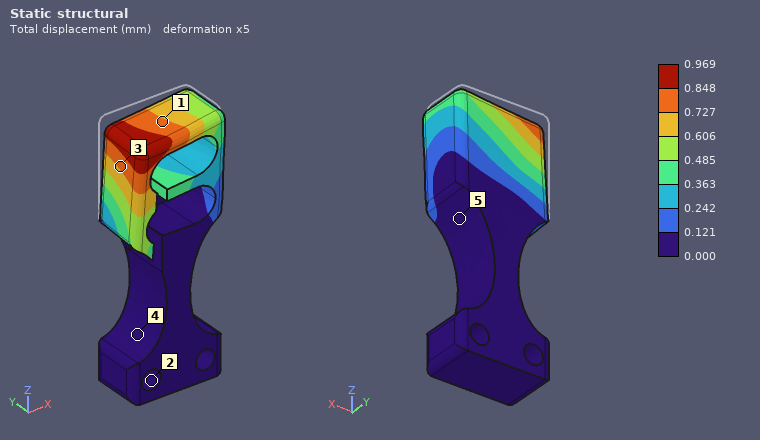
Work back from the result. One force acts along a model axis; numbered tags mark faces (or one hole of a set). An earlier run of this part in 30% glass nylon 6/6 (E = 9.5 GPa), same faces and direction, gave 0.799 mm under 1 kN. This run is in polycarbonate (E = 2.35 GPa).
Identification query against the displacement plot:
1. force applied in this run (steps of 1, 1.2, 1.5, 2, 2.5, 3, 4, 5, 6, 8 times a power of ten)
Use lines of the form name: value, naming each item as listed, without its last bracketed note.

force applied in this run: 300 N
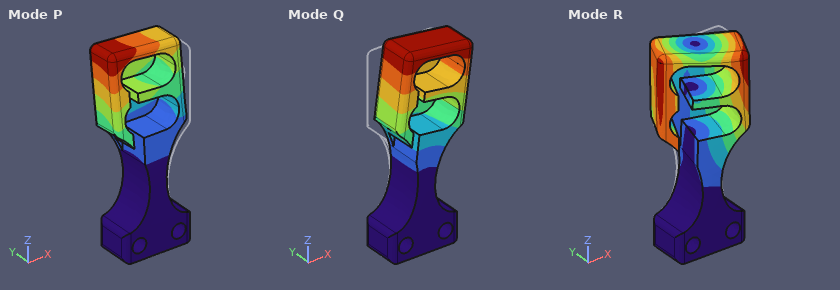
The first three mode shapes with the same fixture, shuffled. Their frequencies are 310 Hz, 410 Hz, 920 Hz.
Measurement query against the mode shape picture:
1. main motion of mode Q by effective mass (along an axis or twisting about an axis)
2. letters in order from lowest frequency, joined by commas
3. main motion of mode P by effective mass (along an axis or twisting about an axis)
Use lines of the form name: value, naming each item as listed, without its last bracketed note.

main motion of mode Q by effective mass: along X
letters in order from lowest frequency, joined by commas: Q, P, R
main motion of mode P by effective mass: along Y
